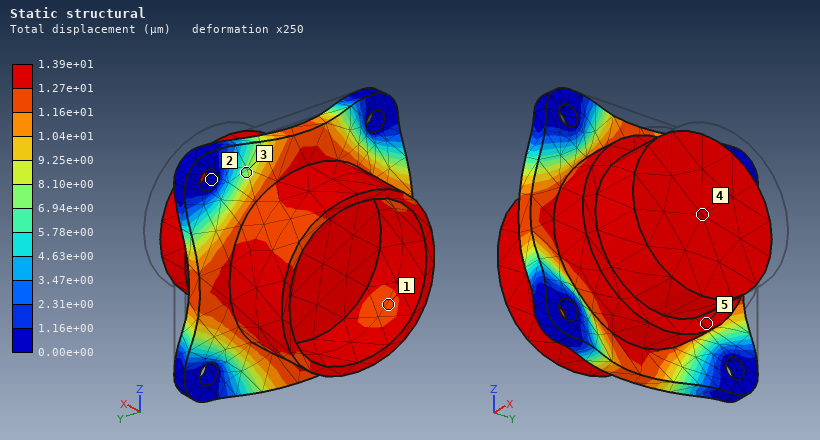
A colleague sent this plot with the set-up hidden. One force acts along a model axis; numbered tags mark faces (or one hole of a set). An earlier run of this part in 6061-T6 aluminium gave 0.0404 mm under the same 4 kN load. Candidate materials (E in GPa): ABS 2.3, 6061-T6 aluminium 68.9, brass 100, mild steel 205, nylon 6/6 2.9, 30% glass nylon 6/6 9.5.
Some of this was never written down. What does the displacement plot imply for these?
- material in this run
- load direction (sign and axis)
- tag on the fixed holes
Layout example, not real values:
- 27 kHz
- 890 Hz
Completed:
- mild steel
- -X
- 2
